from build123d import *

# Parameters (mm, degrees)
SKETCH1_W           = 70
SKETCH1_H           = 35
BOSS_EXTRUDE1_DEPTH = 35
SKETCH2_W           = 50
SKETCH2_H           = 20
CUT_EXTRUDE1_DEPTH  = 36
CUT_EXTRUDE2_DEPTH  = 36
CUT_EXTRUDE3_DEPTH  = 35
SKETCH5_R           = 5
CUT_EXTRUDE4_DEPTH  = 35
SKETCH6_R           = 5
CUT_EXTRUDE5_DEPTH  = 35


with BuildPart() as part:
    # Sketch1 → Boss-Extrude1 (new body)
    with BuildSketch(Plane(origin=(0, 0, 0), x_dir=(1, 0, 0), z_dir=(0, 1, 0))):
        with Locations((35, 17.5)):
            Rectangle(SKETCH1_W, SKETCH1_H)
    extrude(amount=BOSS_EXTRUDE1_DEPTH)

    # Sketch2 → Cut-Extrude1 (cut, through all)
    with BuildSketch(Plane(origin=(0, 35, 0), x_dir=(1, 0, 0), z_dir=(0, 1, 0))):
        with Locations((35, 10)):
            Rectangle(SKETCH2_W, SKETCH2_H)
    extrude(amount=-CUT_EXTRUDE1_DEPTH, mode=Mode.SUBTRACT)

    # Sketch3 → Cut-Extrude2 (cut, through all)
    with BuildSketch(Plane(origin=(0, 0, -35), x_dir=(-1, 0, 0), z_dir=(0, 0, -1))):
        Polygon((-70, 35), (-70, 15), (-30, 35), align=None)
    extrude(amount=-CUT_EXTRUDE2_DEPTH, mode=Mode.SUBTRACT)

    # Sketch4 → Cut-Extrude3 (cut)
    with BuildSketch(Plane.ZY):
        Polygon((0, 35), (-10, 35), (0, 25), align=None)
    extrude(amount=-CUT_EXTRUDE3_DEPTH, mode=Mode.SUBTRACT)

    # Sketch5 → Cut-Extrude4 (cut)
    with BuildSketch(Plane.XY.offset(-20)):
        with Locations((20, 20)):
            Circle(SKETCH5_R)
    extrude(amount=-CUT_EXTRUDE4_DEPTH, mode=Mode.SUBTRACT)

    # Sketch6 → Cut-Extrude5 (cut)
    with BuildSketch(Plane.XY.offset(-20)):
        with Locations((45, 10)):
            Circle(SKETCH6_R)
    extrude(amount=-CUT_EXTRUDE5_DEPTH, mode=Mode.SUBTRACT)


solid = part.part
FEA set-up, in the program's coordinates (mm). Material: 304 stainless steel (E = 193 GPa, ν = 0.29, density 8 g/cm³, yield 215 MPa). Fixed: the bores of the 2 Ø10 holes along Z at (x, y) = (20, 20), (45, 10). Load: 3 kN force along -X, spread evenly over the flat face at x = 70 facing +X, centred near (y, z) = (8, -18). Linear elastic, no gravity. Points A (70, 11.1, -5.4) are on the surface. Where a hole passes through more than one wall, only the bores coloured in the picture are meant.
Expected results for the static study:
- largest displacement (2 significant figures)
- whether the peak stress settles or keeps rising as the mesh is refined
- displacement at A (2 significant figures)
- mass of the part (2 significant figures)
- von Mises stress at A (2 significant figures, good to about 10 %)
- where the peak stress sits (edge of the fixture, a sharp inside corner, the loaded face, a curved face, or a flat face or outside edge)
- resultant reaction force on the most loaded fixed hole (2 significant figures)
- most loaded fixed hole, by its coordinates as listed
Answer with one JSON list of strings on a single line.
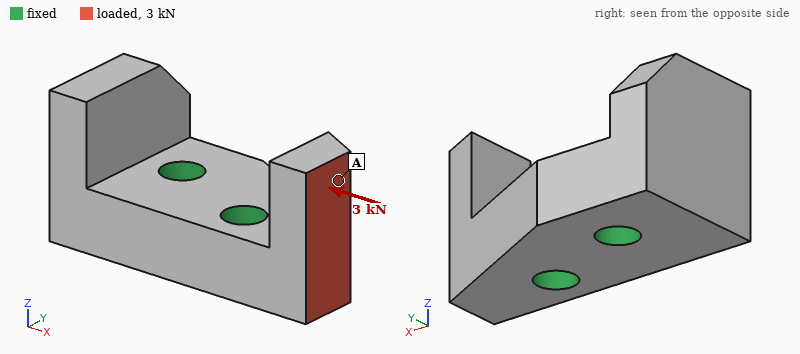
["30 µm", "keeps rising", "23 µm", "310 g", "9.2 MPa", "a sharp inside corner", "2.9 kN", "(45, 10)"]
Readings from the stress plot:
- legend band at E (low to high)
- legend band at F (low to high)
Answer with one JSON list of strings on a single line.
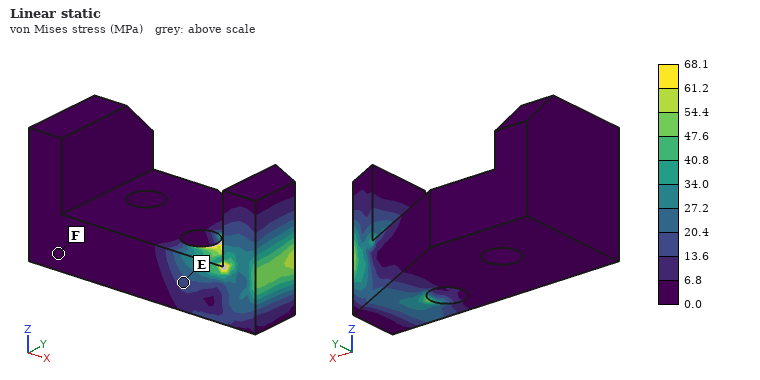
["13.6 to 20.4 MPa", "0.0 to 6.8 MPa"]
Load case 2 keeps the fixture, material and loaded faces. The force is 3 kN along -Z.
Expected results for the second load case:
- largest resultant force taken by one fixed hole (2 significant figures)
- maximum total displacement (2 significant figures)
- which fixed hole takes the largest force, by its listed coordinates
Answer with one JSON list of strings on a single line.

["3.3 kN", "32 µm", "(45, 10)"]
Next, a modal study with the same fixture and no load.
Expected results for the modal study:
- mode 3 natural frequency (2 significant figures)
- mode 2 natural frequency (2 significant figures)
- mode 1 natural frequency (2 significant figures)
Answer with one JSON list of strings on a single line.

["10000 Hz", "9300 Hz", "8500 Hz"]
